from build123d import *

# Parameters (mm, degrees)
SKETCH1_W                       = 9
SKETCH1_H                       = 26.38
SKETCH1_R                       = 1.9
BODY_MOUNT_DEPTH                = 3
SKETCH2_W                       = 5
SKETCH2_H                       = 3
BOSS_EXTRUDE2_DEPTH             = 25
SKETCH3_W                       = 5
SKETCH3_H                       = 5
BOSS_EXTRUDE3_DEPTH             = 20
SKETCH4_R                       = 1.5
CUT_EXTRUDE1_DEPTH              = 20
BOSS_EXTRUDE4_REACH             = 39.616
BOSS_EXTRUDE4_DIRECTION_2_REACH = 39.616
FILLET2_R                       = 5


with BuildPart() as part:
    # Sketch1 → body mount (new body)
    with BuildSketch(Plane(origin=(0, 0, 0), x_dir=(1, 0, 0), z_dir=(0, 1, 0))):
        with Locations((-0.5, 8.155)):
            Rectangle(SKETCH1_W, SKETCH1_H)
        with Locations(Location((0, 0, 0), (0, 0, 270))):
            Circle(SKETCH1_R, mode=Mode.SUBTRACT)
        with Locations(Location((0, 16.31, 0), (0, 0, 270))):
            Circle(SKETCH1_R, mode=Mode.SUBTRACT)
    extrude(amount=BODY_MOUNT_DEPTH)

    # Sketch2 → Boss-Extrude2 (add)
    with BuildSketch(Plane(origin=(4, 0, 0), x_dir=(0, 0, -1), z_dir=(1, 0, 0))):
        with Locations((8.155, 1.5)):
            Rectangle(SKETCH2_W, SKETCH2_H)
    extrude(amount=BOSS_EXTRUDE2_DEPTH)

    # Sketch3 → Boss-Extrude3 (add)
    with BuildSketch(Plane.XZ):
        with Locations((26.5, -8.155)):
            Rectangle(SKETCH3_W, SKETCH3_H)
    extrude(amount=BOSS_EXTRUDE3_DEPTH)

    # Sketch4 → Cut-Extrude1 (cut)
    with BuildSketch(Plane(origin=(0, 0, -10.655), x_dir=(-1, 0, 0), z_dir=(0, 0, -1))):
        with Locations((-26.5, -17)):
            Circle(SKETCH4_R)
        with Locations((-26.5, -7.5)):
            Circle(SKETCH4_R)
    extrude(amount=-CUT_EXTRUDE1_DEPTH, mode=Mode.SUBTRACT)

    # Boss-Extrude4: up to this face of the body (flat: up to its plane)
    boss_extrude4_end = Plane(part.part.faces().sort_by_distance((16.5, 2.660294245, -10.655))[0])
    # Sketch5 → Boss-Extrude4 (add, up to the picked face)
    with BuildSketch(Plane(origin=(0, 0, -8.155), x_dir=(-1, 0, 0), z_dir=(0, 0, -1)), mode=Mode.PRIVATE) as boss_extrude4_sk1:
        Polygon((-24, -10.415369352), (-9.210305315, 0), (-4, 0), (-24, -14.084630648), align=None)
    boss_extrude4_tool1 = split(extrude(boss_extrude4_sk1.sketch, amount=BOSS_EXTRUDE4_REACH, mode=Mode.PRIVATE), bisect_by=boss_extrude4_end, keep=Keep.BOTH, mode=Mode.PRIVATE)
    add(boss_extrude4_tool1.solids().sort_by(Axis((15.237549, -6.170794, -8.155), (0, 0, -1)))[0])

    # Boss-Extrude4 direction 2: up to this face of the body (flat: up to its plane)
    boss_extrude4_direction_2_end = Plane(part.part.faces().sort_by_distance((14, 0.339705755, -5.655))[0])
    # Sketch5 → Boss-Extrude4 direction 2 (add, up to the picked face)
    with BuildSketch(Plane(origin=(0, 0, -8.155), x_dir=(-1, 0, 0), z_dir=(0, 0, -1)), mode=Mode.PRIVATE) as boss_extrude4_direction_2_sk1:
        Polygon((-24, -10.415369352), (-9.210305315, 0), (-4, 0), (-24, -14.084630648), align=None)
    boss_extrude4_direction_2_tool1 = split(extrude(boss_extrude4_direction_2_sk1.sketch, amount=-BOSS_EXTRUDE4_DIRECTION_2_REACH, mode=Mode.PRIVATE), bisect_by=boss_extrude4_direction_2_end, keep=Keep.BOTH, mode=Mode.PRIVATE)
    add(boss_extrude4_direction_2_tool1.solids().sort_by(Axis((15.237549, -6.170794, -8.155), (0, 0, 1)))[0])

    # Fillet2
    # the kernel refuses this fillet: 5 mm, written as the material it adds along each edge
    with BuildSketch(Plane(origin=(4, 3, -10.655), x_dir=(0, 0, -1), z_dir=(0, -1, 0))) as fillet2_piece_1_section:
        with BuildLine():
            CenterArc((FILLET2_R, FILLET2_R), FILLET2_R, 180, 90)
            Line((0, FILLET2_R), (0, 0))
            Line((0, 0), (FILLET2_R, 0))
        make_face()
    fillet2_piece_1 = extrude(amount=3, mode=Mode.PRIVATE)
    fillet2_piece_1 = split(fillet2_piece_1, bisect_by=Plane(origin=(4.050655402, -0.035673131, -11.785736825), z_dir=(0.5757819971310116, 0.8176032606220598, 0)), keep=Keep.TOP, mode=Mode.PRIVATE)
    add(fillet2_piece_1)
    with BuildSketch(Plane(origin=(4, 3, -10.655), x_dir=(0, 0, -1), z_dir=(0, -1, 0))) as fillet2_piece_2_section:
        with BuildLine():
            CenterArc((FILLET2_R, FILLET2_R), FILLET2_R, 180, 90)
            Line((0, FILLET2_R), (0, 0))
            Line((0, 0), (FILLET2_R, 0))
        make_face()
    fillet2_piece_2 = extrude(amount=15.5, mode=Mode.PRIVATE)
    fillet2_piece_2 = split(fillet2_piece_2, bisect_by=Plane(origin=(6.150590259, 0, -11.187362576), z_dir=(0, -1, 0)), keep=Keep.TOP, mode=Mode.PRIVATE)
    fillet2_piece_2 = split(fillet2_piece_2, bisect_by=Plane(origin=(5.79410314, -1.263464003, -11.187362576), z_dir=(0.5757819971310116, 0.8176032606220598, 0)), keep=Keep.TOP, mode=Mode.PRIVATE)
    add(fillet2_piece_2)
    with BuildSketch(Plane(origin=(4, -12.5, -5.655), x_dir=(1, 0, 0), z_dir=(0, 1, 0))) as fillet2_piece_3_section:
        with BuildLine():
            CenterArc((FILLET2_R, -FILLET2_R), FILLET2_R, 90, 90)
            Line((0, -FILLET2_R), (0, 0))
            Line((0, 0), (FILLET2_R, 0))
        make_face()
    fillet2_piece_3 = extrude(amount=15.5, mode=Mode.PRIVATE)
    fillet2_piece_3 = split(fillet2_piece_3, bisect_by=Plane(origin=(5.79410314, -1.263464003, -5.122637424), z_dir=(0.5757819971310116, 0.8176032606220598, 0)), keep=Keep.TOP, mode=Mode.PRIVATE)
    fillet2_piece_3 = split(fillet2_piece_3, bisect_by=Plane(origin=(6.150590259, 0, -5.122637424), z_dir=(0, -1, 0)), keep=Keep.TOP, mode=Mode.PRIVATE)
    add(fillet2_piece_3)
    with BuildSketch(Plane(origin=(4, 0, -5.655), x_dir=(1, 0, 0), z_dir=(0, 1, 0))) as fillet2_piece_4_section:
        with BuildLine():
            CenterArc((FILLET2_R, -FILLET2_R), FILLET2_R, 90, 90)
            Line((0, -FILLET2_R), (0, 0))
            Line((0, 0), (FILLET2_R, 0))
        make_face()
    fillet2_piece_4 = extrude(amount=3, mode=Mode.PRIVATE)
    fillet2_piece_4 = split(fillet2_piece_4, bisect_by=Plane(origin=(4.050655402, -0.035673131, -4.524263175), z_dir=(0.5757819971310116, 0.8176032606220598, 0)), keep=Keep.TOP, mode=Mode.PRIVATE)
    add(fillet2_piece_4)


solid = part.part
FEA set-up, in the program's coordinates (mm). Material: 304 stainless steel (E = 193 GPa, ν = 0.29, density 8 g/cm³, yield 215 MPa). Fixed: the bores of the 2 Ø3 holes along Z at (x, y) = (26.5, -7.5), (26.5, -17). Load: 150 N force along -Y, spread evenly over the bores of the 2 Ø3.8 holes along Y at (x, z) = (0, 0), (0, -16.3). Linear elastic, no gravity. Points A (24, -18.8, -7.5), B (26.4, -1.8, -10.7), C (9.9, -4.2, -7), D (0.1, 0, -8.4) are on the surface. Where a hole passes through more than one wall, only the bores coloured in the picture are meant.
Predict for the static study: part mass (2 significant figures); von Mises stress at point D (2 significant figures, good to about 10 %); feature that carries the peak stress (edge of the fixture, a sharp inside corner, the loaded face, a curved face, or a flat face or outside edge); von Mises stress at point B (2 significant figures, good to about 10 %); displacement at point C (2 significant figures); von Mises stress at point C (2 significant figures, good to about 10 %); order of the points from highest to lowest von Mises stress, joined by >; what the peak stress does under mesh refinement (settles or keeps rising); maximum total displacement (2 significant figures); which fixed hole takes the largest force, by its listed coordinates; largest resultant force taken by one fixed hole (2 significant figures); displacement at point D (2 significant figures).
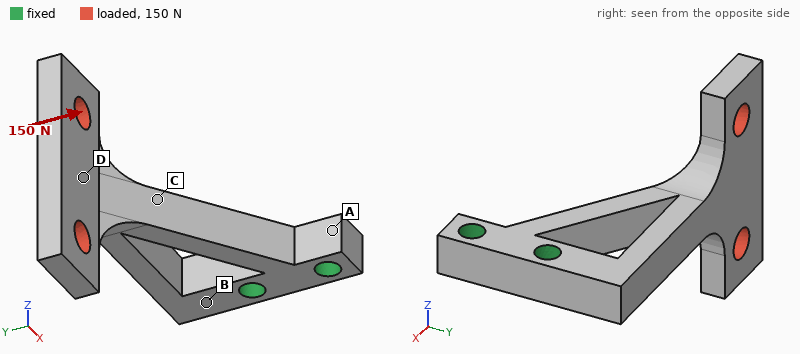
14 g
19 MPa
edge of the fixture
32 MPa
9.0 µm
41 MPa
C > B > D > A
keeps rising
39 µm
(26.5, -17)
250 N
24 µm
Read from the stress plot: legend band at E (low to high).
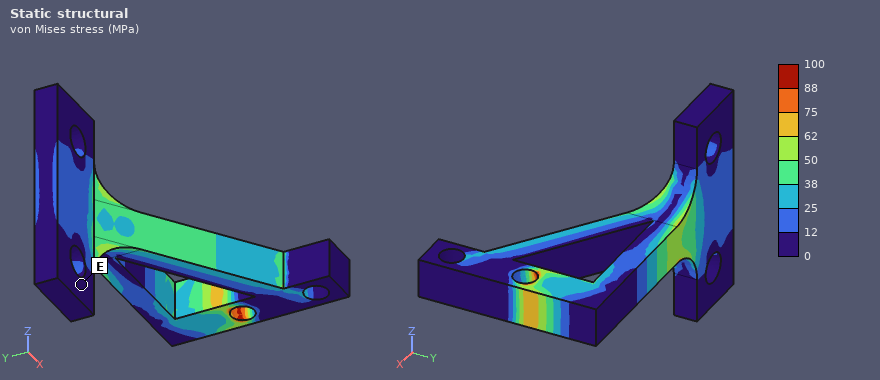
0 to 12 MPa
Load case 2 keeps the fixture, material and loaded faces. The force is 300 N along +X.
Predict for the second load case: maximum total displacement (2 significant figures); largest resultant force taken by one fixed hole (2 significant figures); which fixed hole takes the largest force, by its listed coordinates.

22 µm
360 N
(26.5, -7.5)
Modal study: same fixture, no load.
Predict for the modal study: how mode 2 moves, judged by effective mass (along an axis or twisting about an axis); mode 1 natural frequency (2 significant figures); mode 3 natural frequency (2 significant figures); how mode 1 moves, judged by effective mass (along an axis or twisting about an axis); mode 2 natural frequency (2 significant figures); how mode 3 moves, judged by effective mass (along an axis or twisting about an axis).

along Y
2100 Hz
5200 Hz
along Z
4500 Hz
twisting about X
